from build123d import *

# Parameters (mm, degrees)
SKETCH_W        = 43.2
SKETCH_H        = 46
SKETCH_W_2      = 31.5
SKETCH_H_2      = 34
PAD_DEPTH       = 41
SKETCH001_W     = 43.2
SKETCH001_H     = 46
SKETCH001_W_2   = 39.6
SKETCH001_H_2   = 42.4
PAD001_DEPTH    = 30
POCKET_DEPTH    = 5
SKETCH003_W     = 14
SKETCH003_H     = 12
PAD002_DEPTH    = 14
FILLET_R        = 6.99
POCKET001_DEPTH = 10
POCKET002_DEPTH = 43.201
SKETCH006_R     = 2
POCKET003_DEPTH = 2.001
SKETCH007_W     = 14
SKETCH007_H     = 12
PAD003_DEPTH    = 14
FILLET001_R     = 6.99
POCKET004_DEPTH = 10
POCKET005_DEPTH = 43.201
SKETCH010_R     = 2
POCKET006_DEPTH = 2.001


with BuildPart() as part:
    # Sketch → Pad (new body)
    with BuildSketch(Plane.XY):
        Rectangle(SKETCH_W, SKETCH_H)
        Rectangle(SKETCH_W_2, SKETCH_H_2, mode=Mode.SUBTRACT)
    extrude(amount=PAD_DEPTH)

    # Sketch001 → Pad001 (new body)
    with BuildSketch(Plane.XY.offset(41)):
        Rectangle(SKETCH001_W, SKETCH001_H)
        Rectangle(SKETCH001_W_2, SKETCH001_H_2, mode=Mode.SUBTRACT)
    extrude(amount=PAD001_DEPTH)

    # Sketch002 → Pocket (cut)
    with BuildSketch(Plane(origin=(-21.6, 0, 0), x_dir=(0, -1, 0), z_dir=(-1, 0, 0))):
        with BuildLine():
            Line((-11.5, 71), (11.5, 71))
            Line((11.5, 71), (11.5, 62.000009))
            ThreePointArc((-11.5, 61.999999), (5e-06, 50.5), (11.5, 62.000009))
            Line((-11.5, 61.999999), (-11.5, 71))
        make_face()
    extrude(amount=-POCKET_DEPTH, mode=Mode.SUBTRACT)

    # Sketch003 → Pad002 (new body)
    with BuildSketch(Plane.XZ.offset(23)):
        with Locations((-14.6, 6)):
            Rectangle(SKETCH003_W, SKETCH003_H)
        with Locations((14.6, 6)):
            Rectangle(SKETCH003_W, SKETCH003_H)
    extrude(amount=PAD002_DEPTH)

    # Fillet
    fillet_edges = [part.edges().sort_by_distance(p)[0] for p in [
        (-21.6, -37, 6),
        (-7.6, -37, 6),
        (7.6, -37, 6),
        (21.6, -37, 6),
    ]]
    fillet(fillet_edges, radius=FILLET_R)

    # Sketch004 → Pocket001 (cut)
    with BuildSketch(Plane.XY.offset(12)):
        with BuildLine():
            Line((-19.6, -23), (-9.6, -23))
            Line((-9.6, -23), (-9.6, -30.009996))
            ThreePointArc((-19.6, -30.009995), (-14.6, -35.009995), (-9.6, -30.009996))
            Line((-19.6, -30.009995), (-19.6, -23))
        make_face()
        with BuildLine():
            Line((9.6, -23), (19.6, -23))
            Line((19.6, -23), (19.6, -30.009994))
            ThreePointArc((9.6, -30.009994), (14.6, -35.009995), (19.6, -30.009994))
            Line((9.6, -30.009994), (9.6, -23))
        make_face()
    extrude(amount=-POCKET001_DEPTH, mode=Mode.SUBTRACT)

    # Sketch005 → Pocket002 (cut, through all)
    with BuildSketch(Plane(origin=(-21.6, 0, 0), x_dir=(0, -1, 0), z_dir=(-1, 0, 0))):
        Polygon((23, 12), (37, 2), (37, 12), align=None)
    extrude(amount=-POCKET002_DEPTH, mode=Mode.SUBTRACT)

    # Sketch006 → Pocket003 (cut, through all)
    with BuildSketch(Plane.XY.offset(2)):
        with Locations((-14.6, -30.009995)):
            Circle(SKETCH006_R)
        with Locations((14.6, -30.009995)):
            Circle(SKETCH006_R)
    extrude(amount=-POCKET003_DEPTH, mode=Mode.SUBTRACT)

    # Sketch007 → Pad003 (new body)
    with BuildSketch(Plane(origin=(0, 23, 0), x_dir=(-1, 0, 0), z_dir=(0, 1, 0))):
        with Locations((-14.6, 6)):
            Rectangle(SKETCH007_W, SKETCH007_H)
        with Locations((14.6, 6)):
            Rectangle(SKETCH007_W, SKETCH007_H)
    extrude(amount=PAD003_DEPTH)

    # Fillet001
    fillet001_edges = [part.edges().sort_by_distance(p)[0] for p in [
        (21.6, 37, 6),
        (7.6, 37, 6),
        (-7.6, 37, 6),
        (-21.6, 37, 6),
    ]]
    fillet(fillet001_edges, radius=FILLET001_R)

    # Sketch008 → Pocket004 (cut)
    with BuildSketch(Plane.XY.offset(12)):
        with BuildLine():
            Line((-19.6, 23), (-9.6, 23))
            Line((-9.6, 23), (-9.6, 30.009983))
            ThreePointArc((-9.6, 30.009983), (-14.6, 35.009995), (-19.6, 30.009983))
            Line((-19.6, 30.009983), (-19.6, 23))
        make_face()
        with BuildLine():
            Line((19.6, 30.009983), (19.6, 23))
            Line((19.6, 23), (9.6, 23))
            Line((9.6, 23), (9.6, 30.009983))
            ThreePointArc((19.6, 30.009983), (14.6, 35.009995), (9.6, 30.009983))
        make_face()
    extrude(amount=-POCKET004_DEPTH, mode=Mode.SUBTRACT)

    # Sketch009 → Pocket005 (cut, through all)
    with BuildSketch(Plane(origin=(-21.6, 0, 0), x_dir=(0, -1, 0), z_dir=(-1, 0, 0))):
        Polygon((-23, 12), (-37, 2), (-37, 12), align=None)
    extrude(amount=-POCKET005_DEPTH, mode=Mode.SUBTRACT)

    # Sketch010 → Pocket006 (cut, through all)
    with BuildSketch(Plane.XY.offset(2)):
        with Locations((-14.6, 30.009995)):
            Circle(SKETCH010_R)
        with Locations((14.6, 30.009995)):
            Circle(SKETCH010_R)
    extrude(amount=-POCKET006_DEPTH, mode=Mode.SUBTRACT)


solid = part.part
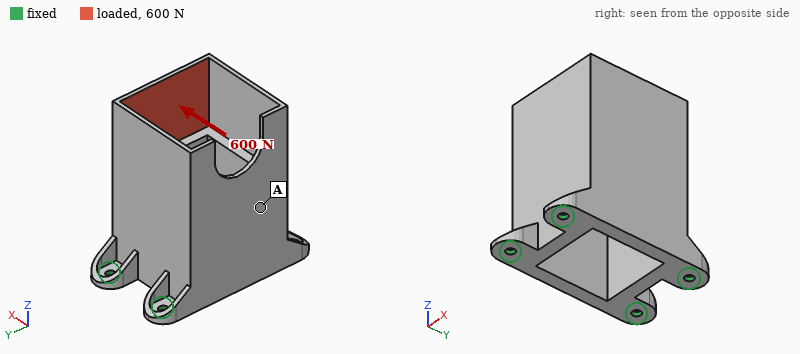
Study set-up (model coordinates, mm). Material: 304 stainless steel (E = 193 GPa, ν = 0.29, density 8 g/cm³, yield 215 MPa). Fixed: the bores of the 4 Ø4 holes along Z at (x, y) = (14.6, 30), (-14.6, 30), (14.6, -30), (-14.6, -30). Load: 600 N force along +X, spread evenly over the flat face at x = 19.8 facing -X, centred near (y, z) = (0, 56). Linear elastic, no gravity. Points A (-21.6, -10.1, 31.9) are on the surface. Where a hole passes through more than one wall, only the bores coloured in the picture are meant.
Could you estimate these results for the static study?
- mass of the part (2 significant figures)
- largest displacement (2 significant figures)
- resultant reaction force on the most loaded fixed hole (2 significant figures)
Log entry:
390 g
0.11 mm
630 N
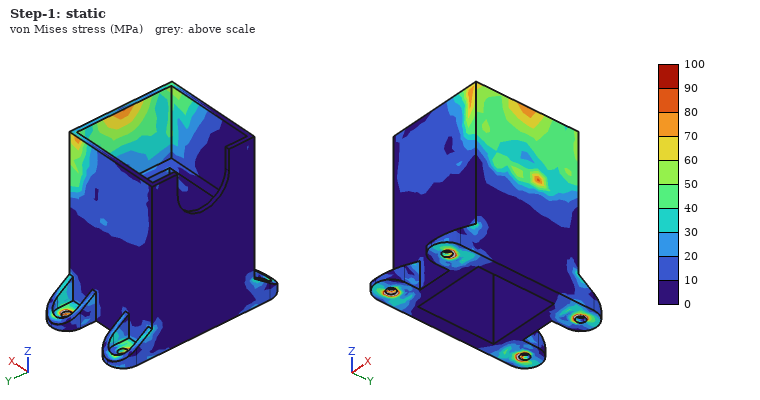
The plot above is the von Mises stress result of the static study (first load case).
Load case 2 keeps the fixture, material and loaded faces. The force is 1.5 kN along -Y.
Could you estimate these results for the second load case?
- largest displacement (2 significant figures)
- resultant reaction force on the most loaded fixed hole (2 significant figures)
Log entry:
40 µm
1.2 kN
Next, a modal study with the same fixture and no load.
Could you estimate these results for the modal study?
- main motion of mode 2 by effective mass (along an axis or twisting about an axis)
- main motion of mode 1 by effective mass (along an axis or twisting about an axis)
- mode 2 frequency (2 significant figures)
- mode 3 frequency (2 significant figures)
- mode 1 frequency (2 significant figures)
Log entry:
along Y
along X
3600 Hz
3700 Hz
2100 Hz
